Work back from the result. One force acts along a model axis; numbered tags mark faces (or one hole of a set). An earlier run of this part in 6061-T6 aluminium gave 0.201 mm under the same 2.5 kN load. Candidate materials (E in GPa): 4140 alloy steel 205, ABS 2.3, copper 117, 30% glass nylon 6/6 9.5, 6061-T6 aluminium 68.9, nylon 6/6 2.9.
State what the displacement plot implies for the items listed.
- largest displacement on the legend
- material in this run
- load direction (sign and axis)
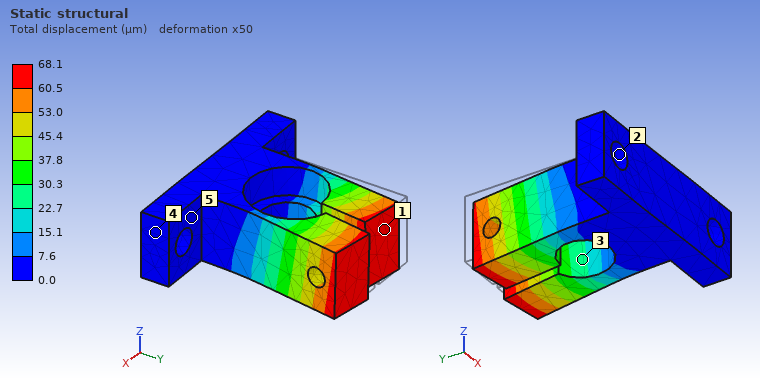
68.1 µm
4140 alloy steel
+X
